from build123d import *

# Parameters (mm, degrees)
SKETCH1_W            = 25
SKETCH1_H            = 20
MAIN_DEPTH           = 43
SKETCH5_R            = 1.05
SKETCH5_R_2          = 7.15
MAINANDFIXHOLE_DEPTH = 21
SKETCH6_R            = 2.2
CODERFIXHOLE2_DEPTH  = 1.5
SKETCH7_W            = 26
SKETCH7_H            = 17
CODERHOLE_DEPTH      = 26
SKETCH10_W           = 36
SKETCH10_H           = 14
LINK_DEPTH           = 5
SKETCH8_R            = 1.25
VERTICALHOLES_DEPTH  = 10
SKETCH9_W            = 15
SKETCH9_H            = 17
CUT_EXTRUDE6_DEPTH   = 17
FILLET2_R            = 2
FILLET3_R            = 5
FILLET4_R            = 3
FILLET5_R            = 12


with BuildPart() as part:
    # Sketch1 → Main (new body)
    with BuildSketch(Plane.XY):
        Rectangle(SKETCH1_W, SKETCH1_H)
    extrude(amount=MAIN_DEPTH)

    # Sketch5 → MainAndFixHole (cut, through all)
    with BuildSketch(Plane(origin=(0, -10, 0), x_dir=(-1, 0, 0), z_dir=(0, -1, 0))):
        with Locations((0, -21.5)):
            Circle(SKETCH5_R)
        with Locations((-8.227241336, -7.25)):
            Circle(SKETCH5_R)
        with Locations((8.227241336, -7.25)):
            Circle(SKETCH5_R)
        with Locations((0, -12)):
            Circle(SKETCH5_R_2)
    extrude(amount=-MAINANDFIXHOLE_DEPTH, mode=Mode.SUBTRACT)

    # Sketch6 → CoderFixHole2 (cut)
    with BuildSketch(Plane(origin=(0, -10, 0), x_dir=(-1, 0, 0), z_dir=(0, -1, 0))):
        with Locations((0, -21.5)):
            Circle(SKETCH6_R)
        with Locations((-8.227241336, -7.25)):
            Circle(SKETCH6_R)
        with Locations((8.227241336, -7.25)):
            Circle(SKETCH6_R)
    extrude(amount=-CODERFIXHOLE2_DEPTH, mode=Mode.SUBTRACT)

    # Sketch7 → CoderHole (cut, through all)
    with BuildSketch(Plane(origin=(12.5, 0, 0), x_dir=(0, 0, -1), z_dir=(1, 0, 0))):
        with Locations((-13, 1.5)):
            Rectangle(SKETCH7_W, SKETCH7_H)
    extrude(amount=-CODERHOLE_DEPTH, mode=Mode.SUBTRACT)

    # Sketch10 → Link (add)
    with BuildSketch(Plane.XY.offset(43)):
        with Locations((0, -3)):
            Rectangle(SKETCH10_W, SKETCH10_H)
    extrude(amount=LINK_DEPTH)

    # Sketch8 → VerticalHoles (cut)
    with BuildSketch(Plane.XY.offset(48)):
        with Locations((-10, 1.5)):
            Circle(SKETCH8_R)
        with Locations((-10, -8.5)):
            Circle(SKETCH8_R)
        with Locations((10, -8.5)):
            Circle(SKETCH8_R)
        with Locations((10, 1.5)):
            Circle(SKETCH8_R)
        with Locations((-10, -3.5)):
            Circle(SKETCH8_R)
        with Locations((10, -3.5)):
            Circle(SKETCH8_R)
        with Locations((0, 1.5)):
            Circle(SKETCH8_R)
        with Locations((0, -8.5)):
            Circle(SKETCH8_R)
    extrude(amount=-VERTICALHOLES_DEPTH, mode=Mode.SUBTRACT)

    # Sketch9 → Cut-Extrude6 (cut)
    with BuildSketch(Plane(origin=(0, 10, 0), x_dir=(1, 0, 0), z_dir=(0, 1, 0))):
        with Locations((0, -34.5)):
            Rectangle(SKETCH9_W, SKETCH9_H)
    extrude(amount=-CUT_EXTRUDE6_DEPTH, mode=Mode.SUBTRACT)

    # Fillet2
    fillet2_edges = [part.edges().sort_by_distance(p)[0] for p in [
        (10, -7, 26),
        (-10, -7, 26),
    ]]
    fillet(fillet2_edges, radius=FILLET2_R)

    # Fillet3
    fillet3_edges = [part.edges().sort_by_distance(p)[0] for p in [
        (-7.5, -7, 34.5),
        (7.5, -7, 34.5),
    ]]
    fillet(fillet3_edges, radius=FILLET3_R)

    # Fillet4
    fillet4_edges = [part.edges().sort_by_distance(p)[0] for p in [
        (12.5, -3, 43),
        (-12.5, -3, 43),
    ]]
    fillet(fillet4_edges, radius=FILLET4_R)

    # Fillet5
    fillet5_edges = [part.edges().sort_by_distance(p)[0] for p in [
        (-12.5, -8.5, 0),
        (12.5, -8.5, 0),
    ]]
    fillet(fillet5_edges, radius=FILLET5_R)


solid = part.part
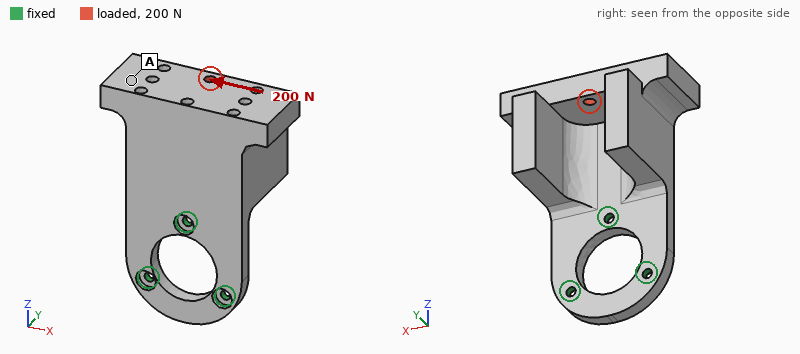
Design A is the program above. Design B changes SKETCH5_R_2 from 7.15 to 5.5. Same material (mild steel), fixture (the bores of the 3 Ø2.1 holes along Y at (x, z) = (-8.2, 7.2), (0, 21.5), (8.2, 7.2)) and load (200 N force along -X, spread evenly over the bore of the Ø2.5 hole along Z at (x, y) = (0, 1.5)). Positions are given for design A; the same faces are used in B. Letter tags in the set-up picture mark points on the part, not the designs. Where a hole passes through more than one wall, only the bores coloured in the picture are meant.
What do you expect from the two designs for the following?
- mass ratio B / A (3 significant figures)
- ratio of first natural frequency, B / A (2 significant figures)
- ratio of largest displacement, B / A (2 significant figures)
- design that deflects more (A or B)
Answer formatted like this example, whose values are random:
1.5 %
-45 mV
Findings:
1.03
1.0
0.82
A
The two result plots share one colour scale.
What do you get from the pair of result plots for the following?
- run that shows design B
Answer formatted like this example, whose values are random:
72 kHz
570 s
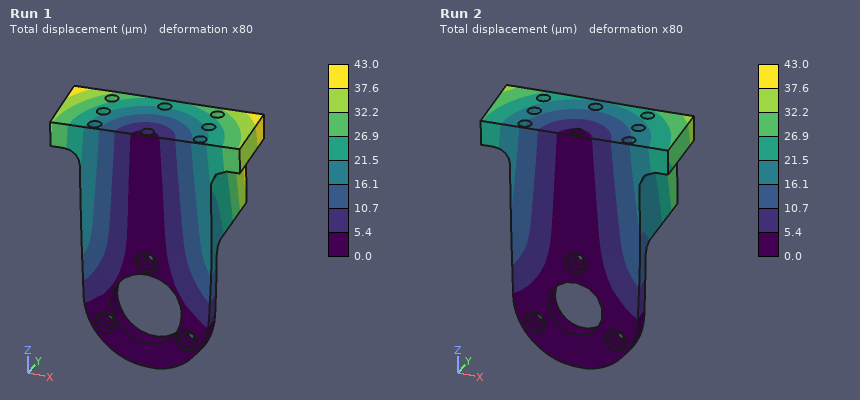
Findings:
Run 2
